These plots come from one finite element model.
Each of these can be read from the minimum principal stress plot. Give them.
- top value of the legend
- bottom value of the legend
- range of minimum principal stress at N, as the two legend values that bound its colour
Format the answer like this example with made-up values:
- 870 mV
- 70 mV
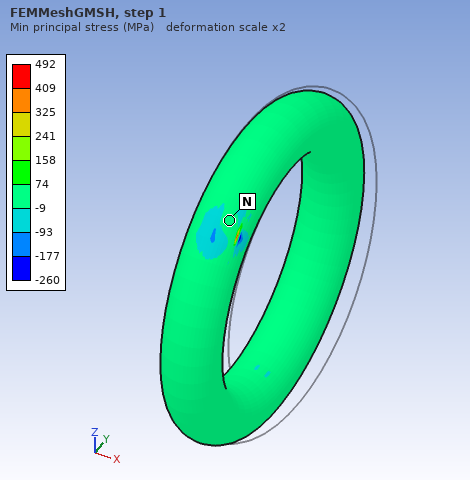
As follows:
- 492 MPa
- -260 MPa
- -9 to 74 MPa
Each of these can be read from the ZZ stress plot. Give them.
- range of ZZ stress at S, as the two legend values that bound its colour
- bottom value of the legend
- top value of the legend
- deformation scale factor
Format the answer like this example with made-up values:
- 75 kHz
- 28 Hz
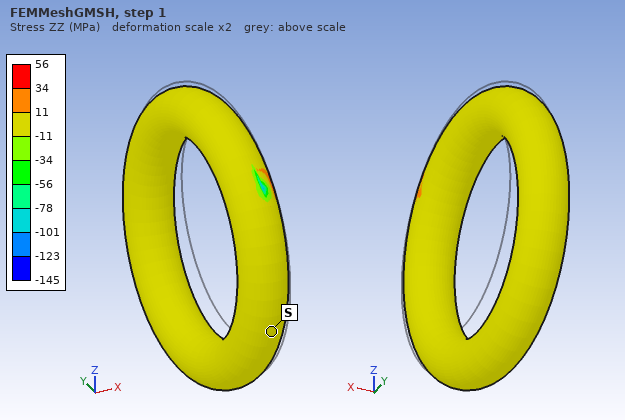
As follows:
- -11 to 11 MPa
- -145 MPa
- 56 MPa
- 2
